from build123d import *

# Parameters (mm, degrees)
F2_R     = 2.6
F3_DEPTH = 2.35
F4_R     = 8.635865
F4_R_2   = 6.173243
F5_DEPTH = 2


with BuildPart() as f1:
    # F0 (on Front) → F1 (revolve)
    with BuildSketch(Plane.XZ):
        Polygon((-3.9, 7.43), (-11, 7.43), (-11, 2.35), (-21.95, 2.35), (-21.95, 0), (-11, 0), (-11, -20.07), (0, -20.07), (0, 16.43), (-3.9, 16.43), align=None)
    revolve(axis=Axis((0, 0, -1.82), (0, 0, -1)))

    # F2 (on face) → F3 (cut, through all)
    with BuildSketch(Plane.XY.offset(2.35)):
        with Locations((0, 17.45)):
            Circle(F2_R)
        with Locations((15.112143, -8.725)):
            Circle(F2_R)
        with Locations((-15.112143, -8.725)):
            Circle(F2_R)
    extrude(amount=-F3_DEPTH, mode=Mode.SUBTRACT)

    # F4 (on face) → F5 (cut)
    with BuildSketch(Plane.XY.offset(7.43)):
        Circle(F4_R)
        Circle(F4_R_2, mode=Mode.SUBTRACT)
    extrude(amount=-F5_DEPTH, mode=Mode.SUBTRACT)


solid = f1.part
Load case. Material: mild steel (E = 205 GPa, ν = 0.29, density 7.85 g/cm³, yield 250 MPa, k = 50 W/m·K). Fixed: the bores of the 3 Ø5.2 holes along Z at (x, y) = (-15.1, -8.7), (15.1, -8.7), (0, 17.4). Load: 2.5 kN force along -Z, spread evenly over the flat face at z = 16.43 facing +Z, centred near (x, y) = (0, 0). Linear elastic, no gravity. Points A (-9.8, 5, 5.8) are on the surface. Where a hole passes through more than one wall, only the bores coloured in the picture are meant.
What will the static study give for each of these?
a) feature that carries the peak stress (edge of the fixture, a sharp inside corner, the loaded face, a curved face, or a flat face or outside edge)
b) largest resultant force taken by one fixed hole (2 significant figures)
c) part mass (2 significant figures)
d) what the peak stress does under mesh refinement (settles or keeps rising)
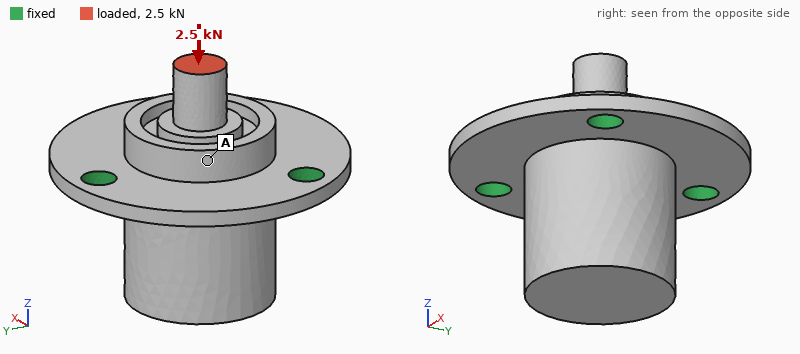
edge of the fixture
830 N
100 g
keeps rising
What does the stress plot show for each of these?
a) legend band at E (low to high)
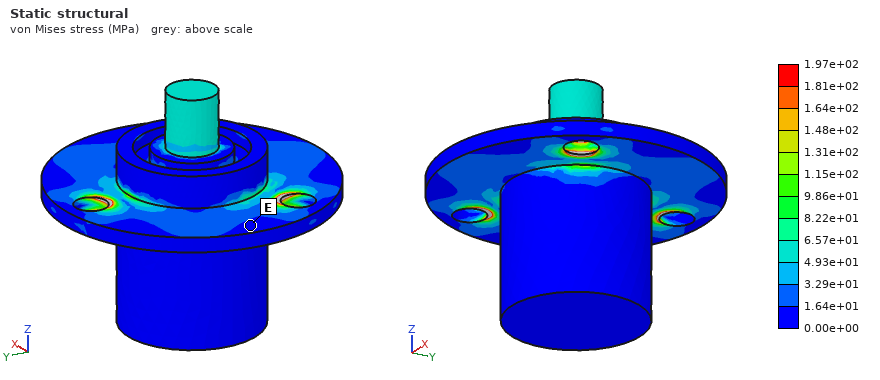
0.00e+00 to 1.64e+01 MPa
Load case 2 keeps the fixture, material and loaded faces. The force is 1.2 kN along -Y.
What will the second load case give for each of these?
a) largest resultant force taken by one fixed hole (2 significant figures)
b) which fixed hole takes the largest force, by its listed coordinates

960 N
(0, 17.4)
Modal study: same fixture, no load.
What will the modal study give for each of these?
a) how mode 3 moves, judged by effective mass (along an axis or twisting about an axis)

along Z
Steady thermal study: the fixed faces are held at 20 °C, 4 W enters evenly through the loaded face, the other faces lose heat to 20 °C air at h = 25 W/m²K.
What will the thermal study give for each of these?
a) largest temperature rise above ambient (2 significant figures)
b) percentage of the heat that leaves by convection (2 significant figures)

24 K
13 %
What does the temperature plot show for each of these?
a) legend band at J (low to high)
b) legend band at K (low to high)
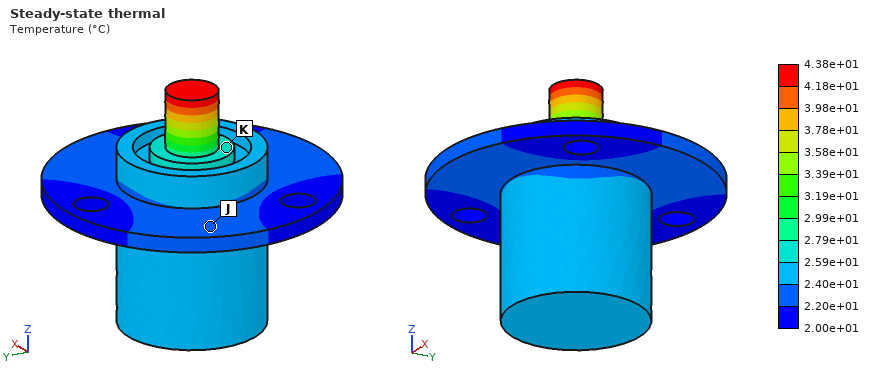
2.20e+01 to 2.40e+01 °C
2.59e+01 to 2.79e+01 °C
